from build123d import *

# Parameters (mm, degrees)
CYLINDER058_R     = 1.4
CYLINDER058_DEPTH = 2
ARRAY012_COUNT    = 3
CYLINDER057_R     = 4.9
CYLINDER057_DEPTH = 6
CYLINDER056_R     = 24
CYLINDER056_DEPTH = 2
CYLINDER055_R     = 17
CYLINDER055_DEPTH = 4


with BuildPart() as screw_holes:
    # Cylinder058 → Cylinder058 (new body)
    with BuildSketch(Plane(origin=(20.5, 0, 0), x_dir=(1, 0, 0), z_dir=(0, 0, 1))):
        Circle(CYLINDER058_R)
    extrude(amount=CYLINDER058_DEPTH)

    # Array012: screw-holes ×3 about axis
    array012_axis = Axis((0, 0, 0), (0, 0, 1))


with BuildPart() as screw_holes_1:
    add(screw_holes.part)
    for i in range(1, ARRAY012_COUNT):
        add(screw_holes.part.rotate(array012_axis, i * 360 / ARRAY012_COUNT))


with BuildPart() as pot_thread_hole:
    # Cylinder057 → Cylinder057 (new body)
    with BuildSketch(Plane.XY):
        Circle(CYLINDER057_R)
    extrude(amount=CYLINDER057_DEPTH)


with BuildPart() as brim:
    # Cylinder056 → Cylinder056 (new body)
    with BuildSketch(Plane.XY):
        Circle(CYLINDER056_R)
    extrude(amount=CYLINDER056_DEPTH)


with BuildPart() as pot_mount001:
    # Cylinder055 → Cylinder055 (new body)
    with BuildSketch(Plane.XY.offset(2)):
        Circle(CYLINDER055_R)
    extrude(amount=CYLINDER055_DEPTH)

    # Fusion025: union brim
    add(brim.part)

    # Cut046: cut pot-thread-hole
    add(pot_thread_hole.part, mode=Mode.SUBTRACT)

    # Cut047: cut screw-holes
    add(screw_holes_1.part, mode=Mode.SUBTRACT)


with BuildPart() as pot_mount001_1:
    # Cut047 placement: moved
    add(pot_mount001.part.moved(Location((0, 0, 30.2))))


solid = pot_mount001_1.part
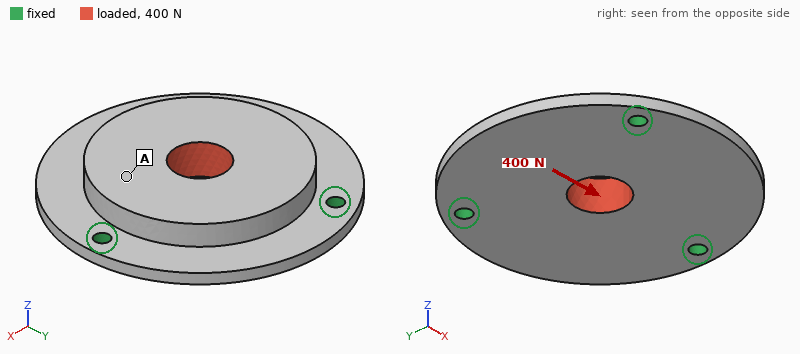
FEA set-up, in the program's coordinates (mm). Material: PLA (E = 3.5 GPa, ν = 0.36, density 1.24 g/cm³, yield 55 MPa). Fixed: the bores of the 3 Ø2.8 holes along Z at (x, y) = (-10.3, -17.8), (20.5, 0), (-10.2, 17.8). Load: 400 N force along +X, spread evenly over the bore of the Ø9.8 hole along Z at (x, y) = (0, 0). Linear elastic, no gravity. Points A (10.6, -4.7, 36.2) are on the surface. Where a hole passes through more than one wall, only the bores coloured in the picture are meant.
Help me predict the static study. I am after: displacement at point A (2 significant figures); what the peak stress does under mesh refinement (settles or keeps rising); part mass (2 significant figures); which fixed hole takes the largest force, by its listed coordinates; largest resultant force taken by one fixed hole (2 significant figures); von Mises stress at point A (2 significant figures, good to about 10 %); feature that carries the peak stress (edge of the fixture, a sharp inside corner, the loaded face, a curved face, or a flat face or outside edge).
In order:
20 µm
keeps rising
8.4 g
(20.5, 0)
160 N
2.2 MPa
edge of the fixture
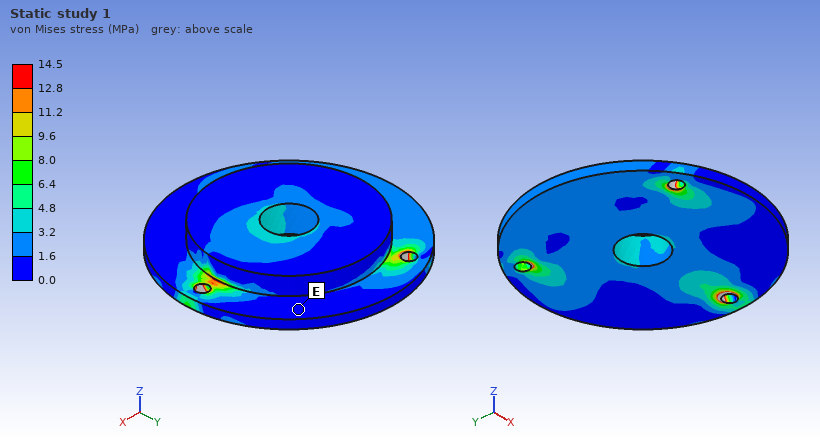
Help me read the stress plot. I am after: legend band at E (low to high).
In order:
0.0 to 1.6 MPa
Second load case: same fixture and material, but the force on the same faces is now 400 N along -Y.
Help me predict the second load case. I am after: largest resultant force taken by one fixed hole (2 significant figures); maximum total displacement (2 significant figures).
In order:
150 N
31 µm
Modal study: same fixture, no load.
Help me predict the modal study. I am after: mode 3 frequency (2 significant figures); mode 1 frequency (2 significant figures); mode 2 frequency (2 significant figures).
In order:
3600 Hz
3400 Hz
3400 Hz
